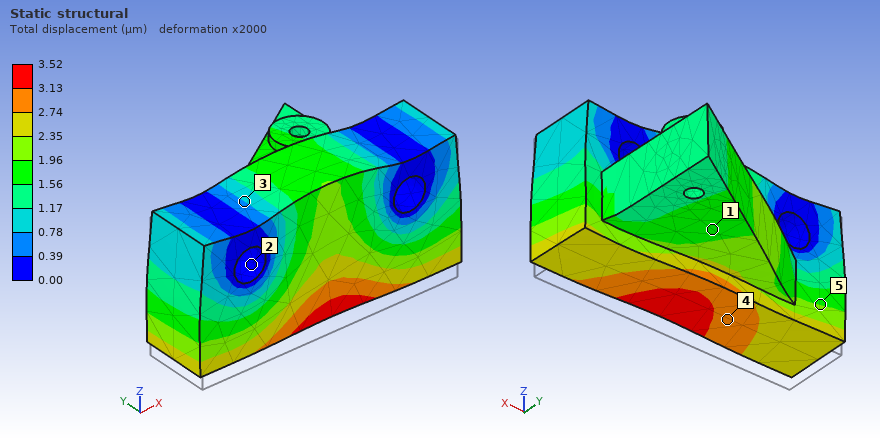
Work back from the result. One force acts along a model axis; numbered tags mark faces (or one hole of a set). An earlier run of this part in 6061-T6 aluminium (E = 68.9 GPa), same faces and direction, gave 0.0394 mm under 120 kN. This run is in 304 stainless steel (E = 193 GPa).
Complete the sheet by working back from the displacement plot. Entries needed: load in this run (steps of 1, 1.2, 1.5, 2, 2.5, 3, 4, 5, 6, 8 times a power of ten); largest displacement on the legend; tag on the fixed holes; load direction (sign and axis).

30 kN
3.52 µm
2
+Z
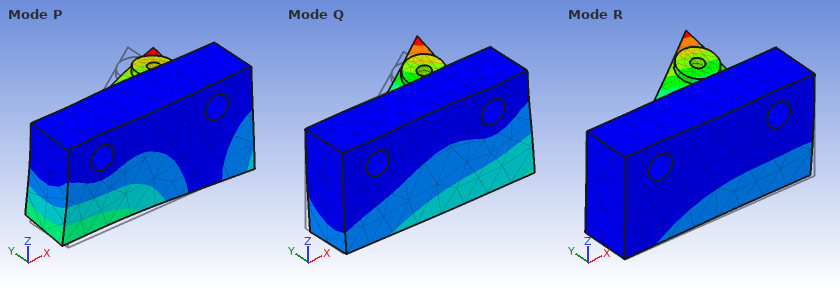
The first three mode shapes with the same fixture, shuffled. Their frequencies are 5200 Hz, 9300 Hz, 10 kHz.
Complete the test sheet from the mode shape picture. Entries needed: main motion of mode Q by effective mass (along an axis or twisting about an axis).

along Y
